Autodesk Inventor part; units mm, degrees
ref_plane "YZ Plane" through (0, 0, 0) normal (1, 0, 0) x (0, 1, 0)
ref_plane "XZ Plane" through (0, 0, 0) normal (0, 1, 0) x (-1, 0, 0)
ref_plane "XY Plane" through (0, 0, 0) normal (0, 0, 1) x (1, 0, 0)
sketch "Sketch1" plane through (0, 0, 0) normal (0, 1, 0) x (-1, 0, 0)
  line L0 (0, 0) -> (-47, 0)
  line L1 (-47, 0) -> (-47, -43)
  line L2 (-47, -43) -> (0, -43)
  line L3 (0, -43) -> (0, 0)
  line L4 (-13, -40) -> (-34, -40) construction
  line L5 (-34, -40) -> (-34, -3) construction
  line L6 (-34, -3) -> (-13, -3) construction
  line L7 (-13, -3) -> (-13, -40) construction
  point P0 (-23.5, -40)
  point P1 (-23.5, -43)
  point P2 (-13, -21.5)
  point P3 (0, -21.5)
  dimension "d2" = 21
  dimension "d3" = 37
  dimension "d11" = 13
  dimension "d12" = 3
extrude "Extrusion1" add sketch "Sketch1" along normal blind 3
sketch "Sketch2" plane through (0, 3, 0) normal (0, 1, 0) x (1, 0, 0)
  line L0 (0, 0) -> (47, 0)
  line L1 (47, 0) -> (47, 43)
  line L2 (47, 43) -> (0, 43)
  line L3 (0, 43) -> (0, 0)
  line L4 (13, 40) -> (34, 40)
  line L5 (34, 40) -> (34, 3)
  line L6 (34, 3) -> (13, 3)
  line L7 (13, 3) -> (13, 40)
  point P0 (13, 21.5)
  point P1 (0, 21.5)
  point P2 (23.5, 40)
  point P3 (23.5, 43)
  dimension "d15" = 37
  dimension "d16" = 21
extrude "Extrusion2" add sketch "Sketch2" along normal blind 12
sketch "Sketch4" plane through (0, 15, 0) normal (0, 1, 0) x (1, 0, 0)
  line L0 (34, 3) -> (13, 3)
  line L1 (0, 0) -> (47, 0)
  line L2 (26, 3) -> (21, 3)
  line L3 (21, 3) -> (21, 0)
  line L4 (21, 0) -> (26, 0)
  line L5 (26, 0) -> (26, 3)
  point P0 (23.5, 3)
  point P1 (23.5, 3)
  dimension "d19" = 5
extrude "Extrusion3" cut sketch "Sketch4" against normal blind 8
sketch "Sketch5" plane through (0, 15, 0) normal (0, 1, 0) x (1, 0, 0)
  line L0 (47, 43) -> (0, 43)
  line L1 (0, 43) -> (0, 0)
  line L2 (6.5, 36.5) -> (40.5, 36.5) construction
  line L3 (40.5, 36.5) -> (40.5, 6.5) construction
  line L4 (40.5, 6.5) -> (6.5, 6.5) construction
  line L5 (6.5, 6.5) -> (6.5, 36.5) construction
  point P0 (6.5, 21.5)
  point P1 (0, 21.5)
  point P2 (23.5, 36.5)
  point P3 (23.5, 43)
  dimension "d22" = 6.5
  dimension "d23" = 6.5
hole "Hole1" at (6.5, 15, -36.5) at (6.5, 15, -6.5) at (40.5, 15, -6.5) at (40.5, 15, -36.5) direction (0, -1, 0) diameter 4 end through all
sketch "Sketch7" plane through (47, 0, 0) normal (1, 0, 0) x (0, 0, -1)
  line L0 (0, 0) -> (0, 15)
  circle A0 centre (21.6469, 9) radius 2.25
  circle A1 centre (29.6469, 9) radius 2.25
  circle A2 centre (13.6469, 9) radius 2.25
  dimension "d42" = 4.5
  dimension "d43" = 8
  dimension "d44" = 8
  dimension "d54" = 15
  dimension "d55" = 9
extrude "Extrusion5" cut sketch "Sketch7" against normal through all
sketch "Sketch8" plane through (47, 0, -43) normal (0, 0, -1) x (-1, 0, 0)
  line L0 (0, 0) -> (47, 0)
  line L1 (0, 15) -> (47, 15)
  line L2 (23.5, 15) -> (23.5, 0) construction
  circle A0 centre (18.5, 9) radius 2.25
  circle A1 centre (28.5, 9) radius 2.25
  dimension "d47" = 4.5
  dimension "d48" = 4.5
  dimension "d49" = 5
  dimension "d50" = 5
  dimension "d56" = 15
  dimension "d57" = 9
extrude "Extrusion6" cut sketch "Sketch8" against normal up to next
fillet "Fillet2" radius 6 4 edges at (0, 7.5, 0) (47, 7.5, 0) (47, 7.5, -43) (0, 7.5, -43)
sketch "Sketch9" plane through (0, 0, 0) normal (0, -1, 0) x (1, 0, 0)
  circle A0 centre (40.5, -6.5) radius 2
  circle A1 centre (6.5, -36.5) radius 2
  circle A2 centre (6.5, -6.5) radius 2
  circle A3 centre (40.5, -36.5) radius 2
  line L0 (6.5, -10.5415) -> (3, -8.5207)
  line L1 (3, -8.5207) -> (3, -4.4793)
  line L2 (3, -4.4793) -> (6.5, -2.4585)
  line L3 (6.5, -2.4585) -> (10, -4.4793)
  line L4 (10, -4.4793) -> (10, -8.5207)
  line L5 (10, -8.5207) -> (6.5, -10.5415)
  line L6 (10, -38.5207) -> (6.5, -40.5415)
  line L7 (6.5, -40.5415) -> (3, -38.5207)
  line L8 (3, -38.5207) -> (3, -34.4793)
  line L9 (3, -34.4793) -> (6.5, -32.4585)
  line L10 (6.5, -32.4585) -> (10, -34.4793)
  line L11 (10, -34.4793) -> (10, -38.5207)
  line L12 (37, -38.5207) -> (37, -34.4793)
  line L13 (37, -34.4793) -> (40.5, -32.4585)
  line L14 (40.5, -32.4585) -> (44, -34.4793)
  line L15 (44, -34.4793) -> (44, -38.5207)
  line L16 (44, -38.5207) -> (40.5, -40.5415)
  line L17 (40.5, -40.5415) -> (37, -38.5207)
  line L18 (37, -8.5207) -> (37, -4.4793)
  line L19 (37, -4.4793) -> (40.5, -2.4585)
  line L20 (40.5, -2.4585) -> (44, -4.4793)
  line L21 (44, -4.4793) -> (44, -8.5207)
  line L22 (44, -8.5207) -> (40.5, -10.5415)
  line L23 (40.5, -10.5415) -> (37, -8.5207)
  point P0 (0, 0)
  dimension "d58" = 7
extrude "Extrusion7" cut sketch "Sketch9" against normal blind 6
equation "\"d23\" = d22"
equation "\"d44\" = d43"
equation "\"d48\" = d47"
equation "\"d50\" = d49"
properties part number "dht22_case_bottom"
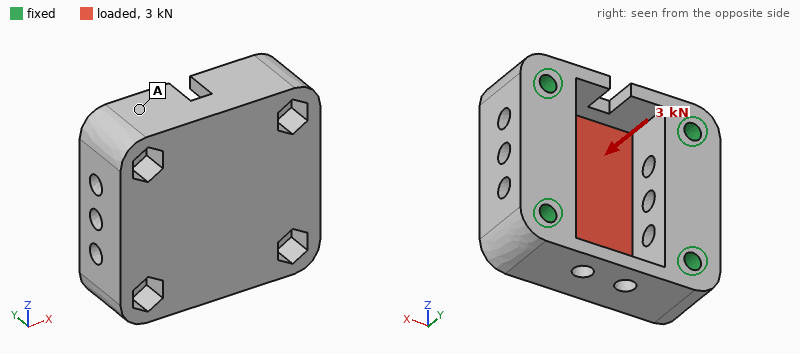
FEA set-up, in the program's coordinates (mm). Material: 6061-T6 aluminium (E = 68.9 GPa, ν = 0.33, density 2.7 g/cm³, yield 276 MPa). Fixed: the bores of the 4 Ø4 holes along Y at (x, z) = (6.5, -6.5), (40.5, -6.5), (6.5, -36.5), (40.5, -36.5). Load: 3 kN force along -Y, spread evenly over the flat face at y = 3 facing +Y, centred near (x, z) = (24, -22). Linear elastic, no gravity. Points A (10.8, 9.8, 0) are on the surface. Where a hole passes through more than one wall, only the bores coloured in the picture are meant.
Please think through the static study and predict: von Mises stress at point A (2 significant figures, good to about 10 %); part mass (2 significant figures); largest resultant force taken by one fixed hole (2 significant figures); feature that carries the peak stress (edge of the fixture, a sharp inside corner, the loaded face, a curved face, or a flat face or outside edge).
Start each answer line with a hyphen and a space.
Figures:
- 10 MPa
- 48 g
- 990 N
- a flat face or outside edge
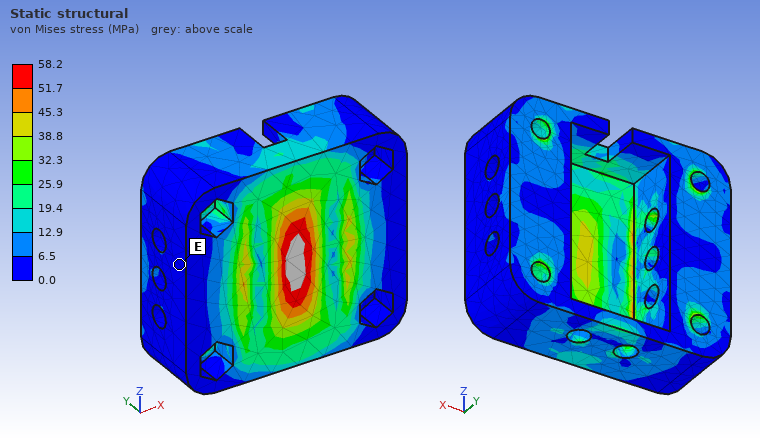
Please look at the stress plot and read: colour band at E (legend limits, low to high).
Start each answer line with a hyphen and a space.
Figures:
- 0.0 to 6.5 MPa
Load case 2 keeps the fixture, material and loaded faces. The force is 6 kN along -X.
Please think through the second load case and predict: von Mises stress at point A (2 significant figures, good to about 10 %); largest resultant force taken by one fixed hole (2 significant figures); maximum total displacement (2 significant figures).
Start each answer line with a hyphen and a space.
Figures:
- 11 MPa
- 1.5 kN
- 15 µm
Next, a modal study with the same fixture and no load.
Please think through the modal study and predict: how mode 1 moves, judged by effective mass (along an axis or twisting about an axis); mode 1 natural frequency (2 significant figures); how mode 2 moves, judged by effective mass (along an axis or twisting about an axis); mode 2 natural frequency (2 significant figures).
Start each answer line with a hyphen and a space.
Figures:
- along Y
- 24 kHz
- along X
- 27 kHz
